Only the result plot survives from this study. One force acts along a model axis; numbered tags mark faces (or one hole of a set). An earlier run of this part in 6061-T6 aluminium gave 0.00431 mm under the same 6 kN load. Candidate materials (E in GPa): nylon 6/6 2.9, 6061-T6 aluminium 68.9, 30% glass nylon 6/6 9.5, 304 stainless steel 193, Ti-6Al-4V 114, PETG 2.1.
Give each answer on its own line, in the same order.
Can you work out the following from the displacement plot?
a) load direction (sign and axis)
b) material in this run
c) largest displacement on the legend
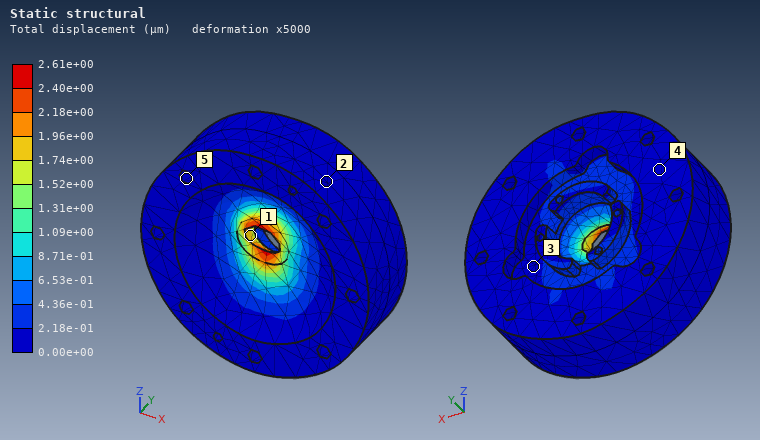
+Z
Ti-6Al-4V
2.61e+00 µm
